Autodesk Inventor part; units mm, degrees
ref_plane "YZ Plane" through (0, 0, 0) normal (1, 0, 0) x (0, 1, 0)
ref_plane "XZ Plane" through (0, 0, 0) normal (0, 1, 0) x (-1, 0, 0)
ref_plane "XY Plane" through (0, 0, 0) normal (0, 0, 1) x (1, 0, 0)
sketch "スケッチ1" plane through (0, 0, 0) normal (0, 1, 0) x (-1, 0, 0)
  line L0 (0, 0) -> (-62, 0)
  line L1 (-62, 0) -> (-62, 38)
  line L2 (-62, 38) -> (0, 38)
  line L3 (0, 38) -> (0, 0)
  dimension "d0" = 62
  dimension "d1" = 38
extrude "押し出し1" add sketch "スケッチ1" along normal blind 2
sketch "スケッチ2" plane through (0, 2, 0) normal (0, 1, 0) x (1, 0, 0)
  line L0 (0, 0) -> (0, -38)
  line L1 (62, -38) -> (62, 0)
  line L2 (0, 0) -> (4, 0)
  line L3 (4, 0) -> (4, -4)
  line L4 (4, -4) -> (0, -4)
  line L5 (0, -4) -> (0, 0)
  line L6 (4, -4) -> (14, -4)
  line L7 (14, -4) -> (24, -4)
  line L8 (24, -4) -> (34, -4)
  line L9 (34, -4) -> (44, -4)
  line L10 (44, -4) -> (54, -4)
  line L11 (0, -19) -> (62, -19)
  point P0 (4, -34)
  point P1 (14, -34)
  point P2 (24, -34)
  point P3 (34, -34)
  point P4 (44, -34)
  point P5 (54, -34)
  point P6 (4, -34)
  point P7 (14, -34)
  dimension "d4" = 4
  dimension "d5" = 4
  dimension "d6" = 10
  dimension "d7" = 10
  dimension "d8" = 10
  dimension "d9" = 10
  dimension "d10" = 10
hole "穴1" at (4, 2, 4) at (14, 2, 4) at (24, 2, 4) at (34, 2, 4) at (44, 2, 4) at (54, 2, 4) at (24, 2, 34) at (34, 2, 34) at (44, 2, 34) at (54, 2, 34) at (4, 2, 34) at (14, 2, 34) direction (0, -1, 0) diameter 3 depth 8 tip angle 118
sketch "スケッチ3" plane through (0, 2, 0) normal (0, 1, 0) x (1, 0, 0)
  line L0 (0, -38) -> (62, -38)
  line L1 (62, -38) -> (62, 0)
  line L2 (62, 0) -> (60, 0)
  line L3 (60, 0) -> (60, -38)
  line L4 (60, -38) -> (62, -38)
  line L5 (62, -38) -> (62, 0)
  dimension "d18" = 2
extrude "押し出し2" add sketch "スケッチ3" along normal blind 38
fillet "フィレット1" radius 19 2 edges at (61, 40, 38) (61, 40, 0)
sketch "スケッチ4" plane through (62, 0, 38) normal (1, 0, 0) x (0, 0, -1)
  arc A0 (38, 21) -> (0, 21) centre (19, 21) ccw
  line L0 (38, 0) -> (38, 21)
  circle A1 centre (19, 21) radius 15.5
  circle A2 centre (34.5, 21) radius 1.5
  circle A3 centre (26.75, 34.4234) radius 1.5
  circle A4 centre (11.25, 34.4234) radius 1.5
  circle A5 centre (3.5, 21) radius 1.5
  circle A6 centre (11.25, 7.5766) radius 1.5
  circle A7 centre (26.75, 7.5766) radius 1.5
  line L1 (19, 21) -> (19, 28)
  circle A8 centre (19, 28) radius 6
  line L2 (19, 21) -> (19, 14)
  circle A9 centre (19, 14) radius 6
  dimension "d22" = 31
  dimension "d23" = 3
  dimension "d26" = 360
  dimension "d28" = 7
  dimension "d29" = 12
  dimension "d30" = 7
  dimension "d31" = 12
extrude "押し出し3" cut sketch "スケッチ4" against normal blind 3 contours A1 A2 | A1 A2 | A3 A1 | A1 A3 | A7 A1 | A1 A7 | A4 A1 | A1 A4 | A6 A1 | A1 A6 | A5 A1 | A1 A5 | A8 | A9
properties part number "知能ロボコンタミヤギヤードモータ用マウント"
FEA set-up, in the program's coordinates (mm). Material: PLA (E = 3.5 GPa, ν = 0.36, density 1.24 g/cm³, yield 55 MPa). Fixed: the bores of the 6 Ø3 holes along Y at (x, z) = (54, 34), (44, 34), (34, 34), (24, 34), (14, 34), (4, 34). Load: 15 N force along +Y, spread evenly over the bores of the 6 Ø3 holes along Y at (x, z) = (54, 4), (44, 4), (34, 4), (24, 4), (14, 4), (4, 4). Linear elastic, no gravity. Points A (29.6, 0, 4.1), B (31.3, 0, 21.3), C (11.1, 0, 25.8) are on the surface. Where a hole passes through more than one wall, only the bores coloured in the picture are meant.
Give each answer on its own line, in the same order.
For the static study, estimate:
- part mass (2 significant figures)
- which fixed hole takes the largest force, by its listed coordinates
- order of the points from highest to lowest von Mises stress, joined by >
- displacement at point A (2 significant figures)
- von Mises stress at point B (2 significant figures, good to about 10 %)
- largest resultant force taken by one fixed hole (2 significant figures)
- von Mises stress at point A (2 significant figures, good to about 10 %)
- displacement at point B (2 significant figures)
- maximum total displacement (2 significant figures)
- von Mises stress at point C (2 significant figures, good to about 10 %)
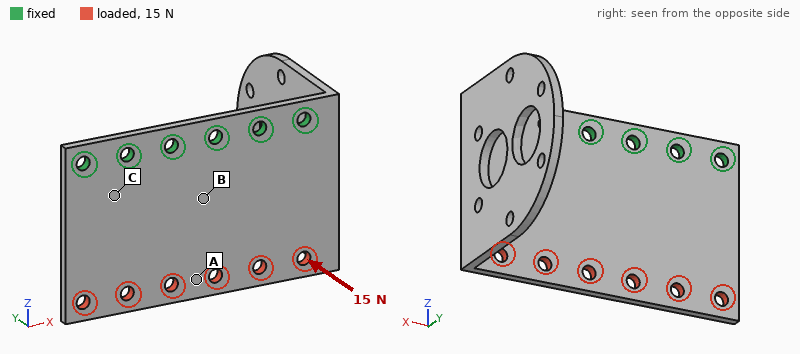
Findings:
8.2 g
(14, 34)
C > B > A
0.66 mm
4.5 MPa
3.7 N
1.7 MPa
0.15 mm
0.92 mm
6.5 MPa
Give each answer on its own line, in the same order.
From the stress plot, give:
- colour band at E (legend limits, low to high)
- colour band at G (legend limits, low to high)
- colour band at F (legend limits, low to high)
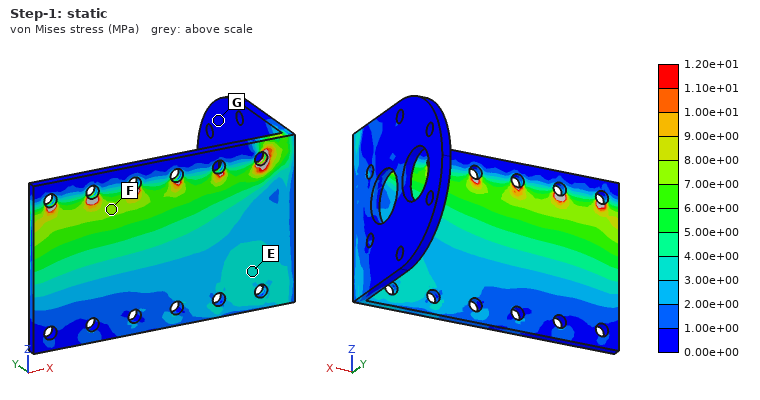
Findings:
3.00e+00 to 4.00e+00 MPa
0.00e+00 to 1.00e+00 MPa
7.00e+00 to 8.00e+00 MPa
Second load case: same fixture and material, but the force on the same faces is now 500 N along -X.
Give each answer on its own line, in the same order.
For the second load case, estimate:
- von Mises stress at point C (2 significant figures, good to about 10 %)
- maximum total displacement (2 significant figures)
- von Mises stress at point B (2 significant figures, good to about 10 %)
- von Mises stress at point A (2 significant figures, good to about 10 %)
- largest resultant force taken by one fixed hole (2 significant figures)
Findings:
8.6 MPa
0.20 mm
10 MPa
7.0 MPa
260 N
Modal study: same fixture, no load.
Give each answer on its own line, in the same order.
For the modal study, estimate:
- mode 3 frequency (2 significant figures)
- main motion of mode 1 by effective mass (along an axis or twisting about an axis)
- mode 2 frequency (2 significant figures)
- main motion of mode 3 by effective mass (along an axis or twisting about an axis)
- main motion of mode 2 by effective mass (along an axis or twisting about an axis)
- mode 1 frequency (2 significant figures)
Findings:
650 Hz
along X
390 Hz
along Y
along Y
290 Hz
